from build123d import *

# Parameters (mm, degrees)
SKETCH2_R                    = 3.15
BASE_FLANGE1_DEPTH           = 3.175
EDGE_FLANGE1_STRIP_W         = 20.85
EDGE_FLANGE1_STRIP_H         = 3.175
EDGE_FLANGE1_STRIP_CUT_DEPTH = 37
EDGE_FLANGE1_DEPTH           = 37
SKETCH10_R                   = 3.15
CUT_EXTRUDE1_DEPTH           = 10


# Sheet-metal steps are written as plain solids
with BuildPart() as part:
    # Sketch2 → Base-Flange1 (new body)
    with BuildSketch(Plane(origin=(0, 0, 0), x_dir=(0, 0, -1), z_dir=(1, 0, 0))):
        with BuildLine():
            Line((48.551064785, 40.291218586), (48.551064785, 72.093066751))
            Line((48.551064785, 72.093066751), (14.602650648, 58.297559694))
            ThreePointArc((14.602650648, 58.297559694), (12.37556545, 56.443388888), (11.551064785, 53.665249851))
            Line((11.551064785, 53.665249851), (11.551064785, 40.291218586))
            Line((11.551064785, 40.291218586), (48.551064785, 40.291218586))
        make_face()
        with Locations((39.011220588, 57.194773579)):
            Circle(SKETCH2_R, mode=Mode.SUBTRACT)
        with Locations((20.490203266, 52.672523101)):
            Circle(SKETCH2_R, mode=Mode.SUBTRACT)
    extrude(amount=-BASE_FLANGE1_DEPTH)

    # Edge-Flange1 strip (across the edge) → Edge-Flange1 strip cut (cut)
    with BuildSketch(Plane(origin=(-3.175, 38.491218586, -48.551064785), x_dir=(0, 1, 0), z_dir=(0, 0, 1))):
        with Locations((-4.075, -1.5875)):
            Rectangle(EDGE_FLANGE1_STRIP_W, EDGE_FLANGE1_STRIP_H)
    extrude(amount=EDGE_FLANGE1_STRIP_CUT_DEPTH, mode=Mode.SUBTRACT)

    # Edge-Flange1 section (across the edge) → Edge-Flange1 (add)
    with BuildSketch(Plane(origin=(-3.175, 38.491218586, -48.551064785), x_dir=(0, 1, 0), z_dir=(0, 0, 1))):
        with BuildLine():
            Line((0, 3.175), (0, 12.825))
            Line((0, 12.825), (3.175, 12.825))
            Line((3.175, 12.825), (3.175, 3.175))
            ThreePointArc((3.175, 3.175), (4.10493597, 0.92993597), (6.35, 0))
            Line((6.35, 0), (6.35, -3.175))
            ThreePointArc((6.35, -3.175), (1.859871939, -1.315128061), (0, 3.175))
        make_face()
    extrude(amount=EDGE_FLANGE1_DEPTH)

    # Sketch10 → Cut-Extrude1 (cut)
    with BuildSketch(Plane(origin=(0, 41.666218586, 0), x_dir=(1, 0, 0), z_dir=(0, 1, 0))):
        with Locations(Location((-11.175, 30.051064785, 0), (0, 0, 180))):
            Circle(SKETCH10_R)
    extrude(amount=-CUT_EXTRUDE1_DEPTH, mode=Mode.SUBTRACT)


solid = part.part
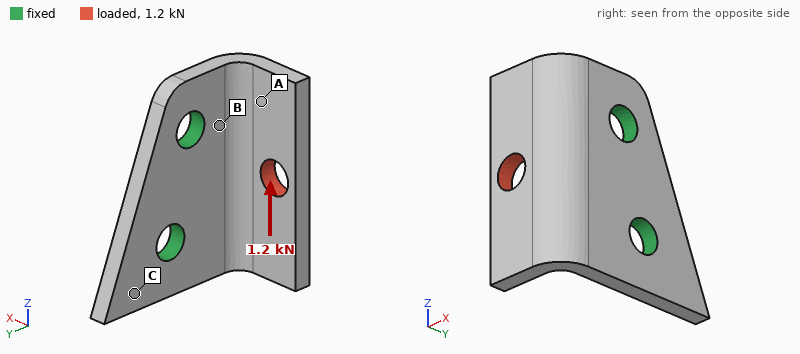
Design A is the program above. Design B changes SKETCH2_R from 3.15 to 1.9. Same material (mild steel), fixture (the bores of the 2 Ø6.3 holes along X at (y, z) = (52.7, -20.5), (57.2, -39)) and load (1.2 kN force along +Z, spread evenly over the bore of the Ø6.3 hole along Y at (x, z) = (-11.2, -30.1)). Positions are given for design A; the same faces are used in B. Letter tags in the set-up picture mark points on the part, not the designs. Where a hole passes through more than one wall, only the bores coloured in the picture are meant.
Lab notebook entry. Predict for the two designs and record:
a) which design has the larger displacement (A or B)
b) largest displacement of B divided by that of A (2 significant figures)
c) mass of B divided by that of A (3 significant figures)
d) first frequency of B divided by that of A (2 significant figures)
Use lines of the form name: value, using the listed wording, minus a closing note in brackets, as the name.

which design has the larger displacement: B
largest displacement of B divided by that of A: 1.2
mass of B divided by that of A: 1.03
first frequency of B divided by that of A: 0.88
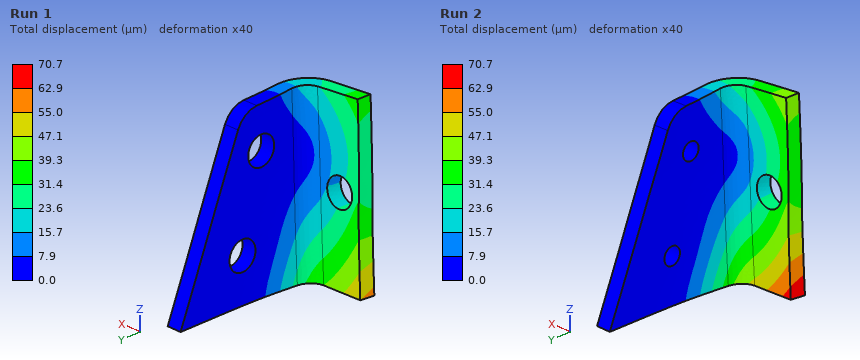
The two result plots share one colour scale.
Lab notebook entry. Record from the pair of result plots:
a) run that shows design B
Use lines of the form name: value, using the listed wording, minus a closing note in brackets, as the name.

run that shows design B: Run 2
